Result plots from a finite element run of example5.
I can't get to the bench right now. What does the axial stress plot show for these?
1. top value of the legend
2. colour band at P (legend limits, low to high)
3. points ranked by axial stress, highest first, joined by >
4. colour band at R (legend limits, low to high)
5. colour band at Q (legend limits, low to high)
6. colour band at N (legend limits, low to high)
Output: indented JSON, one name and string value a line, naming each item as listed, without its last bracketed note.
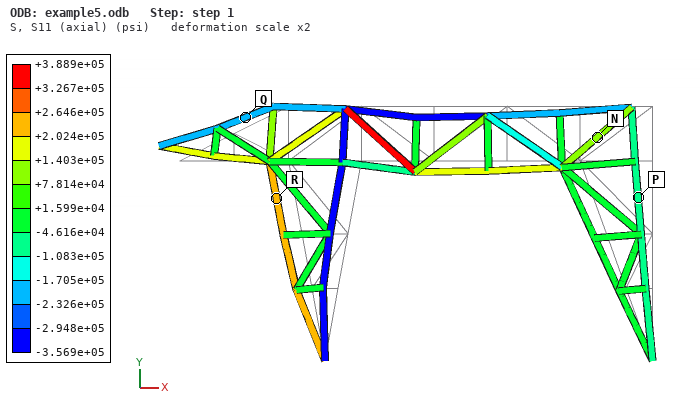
{
  "top value of the legend": "+3.889e+05 psi",
  "colour band at P": "-1.083e+05 to -4.616e+04 psi",
  "points ranked by axial stress, highest first, joined by >": "R > N > P > Q",
  "colour band at R": "+2.024e+05 to +2.646e+05 psi",
  "colour band at Q": "-2.326e+05 to -1.705e+05 psi",
  "colour band at N": "+7.814e+04 to +1.403e+05 psi"
}
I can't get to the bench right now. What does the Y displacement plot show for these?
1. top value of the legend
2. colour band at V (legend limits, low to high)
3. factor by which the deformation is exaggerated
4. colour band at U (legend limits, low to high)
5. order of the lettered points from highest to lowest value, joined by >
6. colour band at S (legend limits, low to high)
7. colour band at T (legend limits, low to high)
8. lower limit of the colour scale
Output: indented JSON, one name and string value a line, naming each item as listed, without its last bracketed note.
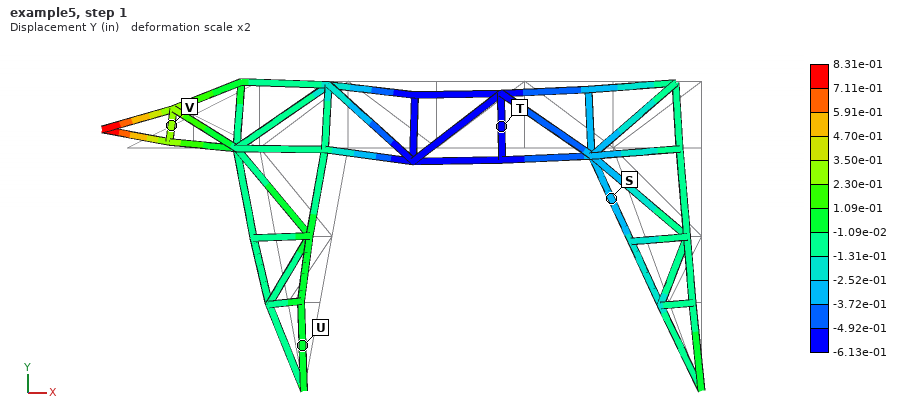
{
  "top value of the legend": "8.31e-01 in",
  "colour band at V": "2.30e-01 to 3.50e-01 in",
  "factor by which the deformation is exaggerated": "2",
  "colour band at U": "-1.09e-02 to 1.09e-01 in",
  "order of the lettered points from highest to lowest value, joined by >": "V > U > S > T",
  "colour band at S": "-3.72e-01 to -2.52e-01 in",
  "colour band at T": "-6.13e-01 to -4.92e-01 in",
  "lower limit of the colour scale": "-6.13e-01 in"
}
